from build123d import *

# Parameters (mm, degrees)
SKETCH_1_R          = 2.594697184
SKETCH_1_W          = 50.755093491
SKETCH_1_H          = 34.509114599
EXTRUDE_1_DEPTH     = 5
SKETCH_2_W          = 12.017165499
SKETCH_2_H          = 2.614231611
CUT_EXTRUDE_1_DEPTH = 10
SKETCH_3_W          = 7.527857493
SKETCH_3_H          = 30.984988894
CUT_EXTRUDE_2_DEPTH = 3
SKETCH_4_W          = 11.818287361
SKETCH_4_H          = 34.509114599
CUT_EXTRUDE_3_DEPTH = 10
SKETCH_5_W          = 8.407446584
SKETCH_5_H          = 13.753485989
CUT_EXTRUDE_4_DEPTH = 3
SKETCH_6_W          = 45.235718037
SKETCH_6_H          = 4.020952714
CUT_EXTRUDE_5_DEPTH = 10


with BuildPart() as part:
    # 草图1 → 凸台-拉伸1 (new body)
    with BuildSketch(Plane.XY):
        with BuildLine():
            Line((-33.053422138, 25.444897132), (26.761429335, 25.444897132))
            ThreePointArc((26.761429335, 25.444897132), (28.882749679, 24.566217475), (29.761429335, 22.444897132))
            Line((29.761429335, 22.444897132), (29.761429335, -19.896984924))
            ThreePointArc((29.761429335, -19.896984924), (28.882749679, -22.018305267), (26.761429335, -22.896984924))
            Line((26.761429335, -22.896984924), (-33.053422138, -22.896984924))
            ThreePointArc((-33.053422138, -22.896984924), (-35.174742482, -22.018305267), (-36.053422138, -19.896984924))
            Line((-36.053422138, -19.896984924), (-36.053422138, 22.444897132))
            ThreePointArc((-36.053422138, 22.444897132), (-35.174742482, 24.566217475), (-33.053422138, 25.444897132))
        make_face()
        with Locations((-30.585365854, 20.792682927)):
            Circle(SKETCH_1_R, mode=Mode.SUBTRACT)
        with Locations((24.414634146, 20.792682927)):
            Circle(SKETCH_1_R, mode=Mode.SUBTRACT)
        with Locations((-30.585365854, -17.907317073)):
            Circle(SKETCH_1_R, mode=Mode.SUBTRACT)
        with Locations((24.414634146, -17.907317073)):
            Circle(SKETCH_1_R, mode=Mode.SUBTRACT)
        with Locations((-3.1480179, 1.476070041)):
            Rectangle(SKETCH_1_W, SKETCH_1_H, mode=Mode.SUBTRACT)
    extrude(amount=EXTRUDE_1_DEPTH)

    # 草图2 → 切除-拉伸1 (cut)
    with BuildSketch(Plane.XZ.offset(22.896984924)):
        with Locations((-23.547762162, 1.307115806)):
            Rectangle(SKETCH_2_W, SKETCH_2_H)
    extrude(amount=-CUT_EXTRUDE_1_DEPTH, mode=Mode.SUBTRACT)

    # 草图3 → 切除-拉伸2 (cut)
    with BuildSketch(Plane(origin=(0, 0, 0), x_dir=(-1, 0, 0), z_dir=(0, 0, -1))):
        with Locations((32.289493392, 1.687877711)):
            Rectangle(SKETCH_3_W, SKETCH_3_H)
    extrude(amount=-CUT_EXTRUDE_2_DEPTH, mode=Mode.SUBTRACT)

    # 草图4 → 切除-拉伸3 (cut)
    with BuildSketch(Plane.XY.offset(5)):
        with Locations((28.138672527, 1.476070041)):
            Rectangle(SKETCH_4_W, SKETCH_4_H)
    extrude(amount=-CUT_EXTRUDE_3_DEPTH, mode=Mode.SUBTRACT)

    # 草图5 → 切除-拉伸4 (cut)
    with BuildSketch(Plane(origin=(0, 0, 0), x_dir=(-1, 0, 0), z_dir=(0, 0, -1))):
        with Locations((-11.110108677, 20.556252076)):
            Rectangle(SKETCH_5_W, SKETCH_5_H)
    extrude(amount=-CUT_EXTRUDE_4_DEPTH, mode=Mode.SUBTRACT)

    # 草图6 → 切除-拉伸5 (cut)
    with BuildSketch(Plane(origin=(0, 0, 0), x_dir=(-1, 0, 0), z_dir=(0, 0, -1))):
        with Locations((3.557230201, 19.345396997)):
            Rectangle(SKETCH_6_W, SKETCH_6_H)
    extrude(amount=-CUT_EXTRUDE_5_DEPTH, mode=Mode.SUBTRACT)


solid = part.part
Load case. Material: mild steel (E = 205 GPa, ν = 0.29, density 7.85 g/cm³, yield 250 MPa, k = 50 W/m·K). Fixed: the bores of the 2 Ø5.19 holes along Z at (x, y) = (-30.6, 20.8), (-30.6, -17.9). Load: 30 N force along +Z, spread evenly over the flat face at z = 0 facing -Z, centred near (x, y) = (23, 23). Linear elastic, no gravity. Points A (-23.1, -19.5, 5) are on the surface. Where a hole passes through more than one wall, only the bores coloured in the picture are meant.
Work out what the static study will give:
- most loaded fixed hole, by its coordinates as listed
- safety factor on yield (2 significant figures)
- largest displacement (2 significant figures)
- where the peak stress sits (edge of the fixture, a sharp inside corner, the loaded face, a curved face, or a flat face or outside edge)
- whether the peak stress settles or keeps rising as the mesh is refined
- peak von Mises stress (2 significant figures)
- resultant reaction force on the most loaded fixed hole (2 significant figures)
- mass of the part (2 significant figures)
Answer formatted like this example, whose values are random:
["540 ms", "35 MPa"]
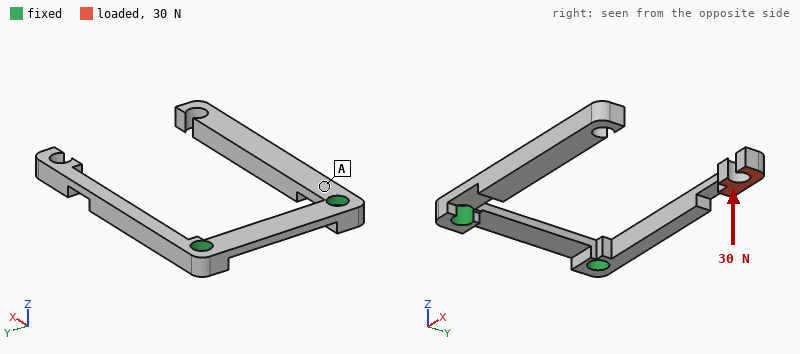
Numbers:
["(-30.6, 20.8)", "1.6", "0.31 mm", "a flat face or outside edge", "settles", "160 MPa", "30 N", "30 g"]
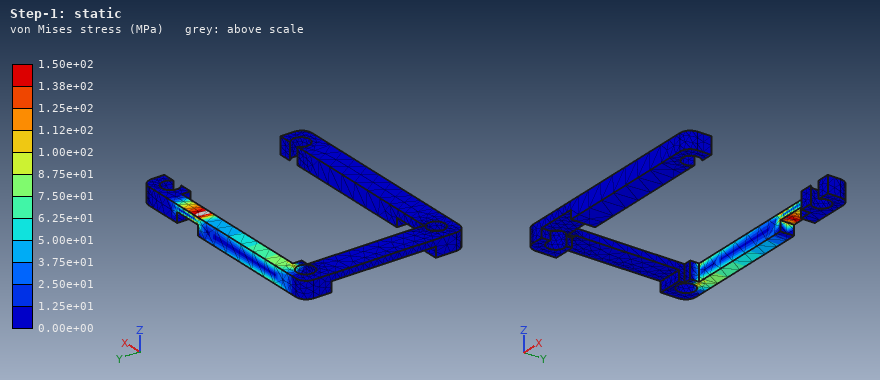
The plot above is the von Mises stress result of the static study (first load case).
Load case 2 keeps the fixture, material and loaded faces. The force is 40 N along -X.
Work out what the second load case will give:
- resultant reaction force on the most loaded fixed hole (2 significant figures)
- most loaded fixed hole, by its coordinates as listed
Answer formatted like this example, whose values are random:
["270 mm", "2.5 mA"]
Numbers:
["40 N", "(-30.6, 20.8)"]
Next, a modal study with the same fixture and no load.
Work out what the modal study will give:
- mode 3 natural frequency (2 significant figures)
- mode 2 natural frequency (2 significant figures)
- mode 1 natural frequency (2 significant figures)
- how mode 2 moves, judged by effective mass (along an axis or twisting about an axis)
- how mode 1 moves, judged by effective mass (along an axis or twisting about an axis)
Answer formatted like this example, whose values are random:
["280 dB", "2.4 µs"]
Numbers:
["1100 Hz", "1000 Hz", "540 Hz", "along Y", "along Z"]
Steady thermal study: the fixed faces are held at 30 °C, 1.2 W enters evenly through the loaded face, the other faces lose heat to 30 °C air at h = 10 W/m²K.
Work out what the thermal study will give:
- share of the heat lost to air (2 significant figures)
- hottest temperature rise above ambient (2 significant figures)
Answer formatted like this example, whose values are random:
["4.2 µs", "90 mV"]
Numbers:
["28 %", "65 K"]
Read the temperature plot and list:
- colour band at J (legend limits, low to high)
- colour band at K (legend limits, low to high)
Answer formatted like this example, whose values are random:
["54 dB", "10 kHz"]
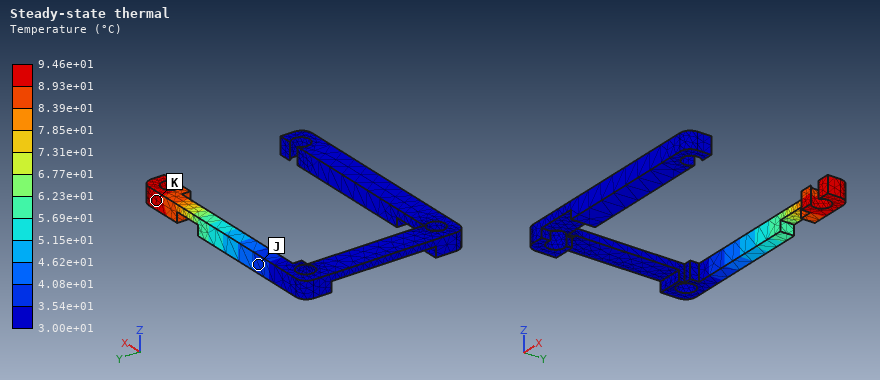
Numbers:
["3.54e+01 to 4.08e+01 °C", "8.93e+01 to 9.46e+01 °C"]
